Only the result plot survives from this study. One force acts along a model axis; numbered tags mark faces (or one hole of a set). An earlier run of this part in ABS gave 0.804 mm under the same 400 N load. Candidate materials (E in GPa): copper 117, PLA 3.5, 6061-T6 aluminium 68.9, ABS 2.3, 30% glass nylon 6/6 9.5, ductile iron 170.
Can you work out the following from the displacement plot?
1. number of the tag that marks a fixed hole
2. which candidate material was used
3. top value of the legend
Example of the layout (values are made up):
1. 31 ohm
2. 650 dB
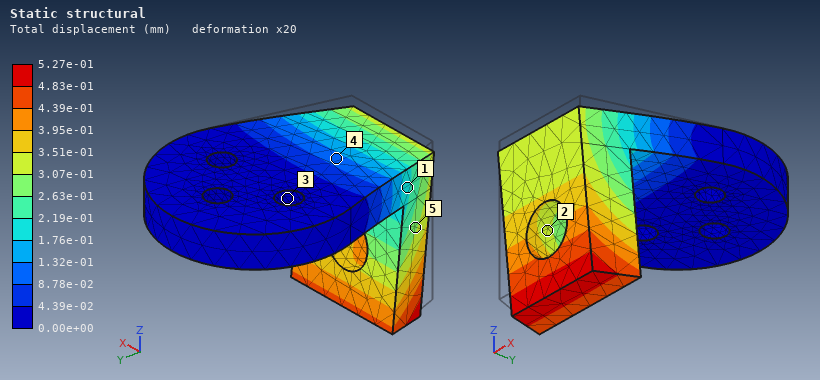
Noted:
1. 3
2. PLA
3. 5.27e-01 mm
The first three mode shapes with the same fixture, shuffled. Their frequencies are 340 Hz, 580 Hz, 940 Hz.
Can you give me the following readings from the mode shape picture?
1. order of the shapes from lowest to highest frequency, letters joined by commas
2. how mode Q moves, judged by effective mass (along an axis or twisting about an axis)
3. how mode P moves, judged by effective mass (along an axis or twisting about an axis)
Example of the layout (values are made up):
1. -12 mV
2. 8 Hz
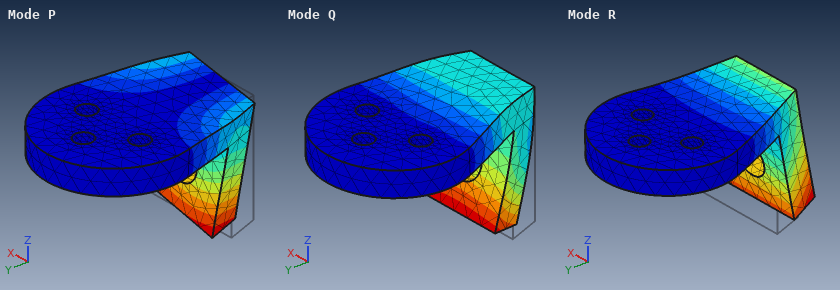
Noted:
1. R, P, Q
2. along Z
3. along X
